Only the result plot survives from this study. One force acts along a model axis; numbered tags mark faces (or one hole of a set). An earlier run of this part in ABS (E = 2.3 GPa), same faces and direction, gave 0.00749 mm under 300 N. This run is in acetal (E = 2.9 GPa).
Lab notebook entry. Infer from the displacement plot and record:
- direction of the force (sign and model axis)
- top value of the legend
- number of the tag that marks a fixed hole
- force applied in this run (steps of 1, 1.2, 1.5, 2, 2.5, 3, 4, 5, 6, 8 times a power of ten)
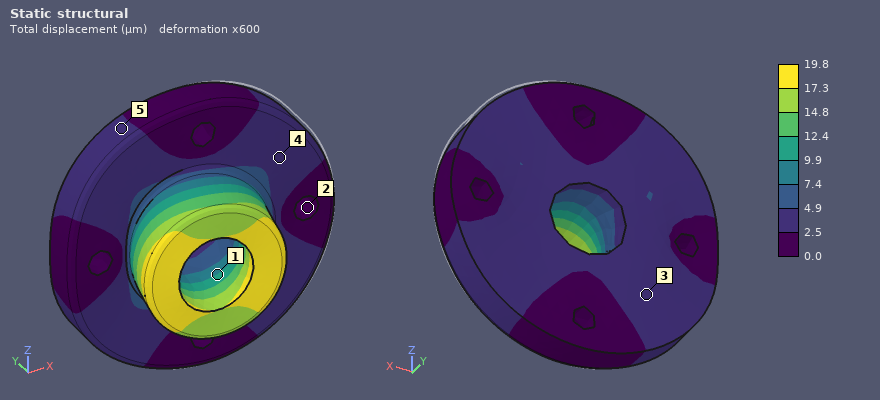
-X
19.8 µm
2
1 kN
